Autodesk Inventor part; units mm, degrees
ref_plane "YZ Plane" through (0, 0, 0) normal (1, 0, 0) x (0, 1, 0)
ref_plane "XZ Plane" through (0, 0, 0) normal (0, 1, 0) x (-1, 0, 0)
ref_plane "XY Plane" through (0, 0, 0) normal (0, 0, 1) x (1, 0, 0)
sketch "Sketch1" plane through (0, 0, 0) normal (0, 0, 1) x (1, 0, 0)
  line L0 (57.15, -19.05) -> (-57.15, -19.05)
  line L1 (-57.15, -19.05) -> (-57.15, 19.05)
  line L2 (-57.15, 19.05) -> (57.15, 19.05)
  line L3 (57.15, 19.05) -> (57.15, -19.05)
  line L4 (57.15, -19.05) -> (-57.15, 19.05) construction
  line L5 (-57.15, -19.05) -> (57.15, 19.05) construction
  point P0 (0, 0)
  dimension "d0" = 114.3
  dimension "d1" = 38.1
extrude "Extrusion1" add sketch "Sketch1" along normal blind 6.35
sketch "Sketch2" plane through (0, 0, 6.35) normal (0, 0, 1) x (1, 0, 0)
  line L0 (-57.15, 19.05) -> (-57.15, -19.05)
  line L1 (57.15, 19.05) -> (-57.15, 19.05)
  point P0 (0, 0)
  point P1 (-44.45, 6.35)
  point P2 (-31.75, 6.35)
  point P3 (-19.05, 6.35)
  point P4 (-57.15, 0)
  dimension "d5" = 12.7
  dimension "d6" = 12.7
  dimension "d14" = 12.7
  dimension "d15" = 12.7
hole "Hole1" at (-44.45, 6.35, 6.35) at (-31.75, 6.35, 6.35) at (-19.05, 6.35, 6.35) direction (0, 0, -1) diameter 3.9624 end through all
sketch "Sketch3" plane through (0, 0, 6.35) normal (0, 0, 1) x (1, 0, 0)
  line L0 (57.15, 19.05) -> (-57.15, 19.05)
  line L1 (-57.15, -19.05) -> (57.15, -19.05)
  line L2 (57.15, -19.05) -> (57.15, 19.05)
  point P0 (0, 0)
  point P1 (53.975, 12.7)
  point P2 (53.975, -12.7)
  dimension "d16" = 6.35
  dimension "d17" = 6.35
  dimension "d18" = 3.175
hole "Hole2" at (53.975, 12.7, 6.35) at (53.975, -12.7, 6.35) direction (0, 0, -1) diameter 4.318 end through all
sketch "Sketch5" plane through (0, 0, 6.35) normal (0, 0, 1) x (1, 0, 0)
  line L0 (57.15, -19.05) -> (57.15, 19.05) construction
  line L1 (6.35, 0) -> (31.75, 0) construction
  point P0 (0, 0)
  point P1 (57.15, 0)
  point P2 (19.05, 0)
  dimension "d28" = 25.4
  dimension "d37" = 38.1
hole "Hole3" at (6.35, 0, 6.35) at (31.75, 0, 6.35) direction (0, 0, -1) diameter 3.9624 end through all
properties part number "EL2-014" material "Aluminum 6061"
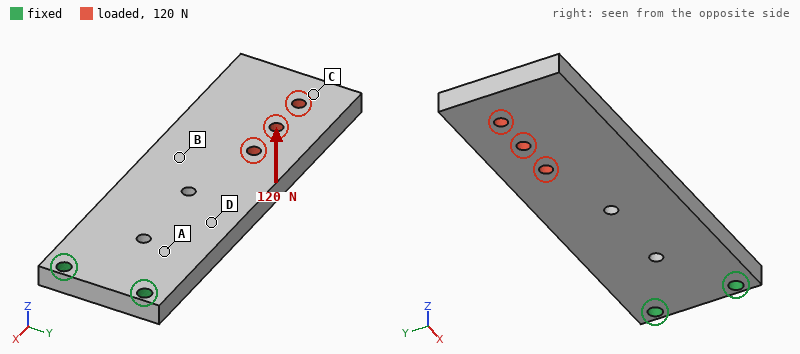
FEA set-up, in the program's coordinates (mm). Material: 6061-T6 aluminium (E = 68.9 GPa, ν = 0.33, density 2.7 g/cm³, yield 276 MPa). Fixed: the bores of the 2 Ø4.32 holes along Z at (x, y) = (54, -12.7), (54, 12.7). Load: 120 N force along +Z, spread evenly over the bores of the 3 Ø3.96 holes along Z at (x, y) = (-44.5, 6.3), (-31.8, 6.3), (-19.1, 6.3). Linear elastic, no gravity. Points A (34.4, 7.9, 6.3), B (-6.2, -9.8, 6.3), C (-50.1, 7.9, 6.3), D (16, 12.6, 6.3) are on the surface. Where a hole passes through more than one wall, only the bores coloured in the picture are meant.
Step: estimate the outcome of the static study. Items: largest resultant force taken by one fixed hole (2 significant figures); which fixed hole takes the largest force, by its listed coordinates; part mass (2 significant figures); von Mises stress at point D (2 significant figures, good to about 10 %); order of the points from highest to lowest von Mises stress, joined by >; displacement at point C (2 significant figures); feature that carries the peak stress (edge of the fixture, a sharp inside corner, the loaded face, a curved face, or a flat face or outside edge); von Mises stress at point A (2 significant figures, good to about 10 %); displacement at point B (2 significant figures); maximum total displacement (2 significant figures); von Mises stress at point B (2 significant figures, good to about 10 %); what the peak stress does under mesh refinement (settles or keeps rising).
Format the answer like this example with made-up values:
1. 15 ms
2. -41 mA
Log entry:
1. 86 N
2. (54, 12.7)
3. 73 g
4. 23 MPa
5. A > D > B > C
6. 0.64 mm
7. edge of the fixture
8. 32 MPa
9. 0.27 mm
10. 0.71 mm
11. 12 MPa
12. keeps rising
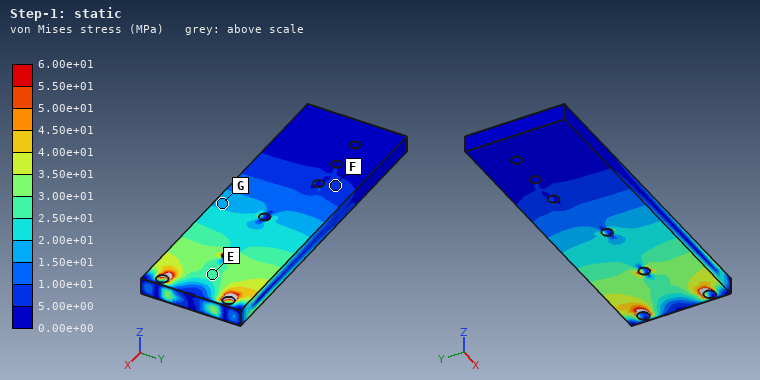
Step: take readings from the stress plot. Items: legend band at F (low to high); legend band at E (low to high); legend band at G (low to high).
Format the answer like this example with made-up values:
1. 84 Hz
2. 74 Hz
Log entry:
1. 5.00e+00 to 1.00e+01 MPa
2. 2.50e+01 to 3.00e+01 MPa
3. 1.50e+01 to 2.00e+01 MPa
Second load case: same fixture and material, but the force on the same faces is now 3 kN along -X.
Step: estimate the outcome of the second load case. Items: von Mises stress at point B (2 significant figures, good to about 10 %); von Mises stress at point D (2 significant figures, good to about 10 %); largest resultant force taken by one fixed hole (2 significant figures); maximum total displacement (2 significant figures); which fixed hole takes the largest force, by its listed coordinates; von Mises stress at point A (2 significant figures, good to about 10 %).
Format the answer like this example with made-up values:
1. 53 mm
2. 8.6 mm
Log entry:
1. 6.2 MPa
2. 21 MPa
3. 2.2 kN
4. 64 µm
5. (54, 12.7)
6. 18 MPa
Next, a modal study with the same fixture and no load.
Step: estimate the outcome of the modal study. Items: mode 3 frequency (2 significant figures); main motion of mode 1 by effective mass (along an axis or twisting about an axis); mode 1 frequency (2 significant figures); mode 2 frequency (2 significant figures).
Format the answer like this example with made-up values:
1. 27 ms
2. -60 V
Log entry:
1. 2300 Hz
2. along Z
3. 410 Hz
4. 2300 Hz
